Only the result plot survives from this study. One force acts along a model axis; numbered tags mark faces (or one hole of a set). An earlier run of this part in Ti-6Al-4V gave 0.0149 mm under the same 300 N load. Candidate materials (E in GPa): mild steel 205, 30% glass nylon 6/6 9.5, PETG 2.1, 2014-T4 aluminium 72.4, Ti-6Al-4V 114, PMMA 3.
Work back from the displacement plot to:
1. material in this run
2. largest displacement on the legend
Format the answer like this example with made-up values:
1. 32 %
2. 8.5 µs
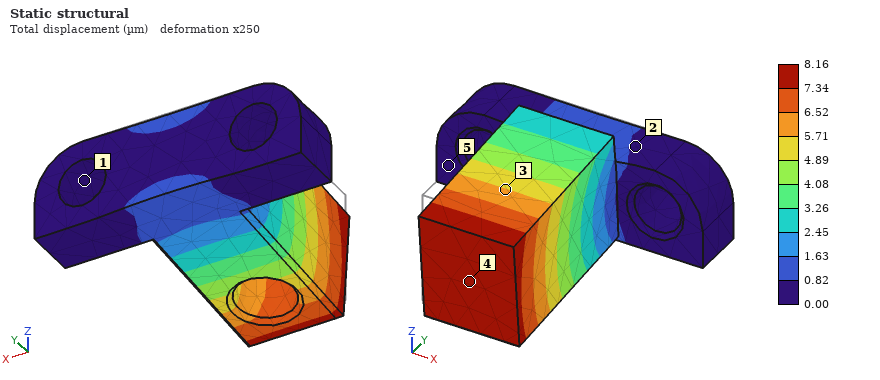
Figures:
1. mild steel
2. 8.16 µm
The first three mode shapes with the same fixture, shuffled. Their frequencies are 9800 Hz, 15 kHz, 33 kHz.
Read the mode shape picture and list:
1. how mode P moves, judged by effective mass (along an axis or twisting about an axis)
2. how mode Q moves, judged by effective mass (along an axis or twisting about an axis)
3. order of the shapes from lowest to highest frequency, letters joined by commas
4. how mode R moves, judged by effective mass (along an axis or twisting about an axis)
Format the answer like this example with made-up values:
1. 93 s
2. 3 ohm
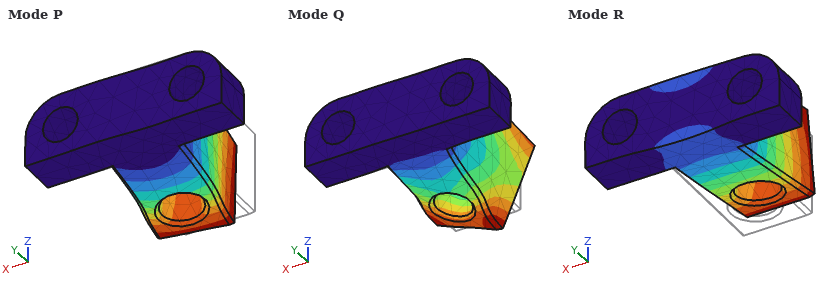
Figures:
1. along X
2. twisting about Y
3. R, P, Q
4. along Z
